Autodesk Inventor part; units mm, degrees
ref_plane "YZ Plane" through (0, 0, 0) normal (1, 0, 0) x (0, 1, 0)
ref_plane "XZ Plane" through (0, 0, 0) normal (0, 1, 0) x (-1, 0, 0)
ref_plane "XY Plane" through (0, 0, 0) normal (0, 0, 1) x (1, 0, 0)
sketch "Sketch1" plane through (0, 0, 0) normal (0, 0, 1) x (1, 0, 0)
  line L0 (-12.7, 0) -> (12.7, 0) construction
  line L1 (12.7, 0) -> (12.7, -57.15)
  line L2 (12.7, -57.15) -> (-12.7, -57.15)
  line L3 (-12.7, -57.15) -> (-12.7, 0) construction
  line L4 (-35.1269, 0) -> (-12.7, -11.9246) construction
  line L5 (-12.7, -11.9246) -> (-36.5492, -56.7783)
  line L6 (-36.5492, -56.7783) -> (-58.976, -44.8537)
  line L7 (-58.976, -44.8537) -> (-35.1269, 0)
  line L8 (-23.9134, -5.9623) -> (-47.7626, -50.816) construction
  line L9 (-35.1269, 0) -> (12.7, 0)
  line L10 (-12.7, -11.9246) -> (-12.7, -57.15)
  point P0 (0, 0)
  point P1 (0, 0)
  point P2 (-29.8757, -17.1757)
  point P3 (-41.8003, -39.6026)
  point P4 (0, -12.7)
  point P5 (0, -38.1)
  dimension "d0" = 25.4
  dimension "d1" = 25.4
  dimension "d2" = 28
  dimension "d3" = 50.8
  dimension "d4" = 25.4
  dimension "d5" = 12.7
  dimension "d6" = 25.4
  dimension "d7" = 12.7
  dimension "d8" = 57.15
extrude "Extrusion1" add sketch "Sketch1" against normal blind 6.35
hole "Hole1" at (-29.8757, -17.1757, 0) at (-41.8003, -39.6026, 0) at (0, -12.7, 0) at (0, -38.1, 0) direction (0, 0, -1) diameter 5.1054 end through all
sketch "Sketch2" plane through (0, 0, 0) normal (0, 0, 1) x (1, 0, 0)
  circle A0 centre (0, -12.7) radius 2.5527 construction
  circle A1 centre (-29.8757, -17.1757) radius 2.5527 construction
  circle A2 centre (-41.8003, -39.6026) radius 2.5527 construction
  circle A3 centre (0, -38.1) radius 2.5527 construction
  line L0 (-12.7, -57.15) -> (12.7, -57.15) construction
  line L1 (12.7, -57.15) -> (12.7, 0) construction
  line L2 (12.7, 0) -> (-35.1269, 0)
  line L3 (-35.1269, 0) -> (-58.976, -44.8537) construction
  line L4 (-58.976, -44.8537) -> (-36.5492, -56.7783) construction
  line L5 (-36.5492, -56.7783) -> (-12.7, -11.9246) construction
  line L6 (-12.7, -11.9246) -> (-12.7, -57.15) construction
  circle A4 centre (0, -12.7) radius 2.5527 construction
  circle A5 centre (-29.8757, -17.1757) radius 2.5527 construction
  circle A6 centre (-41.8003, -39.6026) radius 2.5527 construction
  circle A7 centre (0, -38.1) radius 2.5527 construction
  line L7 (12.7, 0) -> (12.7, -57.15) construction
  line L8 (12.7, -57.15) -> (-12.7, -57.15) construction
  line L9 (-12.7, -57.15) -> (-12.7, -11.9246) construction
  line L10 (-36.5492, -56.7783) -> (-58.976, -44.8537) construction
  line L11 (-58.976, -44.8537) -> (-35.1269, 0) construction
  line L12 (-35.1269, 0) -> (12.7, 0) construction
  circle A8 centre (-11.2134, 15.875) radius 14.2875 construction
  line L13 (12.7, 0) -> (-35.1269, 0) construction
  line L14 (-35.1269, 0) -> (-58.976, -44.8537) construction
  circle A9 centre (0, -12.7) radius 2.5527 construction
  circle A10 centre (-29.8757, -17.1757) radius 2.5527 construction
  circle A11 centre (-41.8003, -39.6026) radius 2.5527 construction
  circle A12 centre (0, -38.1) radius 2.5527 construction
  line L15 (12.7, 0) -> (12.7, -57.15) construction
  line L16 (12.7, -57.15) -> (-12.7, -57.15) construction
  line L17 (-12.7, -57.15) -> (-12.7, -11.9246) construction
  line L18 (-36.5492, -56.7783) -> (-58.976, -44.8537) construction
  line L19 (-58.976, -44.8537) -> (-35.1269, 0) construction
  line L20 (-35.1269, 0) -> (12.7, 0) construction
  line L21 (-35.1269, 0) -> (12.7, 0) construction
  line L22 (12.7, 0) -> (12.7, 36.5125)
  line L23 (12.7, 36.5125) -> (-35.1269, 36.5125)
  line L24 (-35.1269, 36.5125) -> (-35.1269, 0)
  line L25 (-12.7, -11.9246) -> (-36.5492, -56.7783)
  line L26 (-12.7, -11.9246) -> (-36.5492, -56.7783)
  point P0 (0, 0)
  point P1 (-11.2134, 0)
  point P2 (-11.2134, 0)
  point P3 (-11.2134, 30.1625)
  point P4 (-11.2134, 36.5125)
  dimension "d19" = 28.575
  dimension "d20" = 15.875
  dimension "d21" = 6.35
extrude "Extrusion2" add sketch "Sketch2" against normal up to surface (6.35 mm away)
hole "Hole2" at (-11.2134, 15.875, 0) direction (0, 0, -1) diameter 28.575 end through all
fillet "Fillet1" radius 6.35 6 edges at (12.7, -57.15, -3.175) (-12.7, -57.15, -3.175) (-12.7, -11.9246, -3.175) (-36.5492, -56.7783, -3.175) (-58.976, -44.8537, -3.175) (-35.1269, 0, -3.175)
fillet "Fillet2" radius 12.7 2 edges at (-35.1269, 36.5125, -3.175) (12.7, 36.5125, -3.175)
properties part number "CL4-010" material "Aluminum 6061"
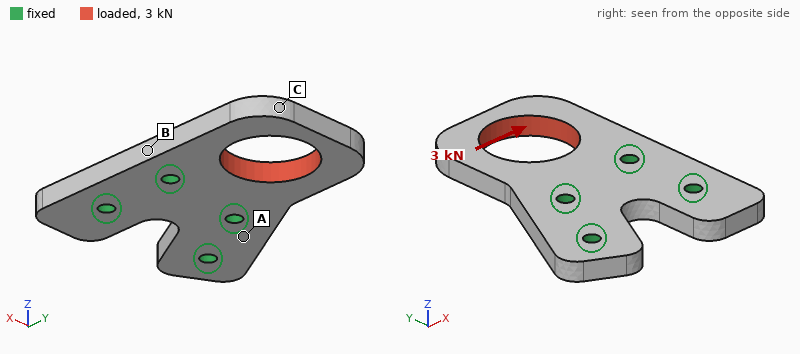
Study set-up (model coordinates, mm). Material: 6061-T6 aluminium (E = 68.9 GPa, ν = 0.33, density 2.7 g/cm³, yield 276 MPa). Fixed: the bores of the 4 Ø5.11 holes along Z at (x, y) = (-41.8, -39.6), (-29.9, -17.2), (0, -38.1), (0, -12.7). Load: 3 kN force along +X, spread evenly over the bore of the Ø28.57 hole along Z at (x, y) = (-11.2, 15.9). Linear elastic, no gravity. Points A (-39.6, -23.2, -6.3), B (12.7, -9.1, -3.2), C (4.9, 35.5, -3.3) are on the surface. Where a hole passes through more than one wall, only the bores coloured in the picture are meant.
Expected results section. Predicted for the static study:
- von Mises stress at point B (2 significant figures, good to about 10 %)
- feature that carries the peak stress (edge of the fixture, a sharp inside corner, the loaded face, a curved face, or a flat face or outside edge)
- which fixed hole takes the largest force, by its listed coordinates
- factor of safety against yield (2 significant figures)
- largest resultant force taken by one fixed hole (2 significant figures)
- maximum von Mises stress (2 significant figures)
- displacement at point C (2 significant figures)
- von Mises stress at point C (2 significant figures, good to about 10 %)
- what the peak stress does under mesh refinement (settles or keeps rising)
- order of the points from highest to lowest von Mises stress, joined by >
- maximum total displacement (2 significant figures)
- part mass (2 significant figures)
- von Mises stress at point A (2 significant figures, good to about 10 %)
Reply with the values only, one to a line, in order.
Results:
42 MPa
the loaded face
(0, -12.7)
3.3
2.7 kN
83 MPa
83 µm
23 MPa
settles
B > C > A
83 µm
67 g
9.7 MPa
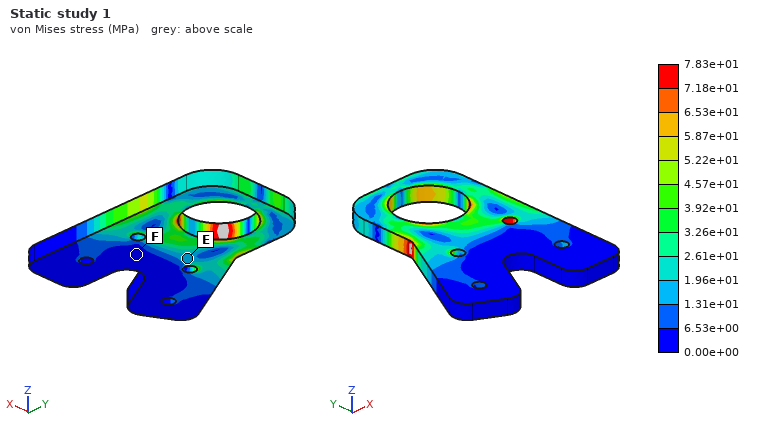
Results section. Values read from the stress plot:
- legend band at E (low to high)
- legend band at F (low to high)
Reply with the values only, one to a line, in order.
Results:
1.31e+01 to 1.96e+01 MPa
0.00e+00 to 6.53e+00 MPa
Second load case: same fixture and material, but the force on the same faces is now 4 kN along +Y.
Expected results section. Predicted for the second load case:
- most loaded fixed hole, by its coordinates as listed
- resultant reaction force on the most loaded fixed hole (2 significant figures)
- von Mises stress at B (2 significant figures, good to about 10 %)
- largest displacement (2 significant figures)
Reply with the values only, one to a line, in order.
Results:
(0, -12.7)
1.9 kN
20 MPa
28 µm
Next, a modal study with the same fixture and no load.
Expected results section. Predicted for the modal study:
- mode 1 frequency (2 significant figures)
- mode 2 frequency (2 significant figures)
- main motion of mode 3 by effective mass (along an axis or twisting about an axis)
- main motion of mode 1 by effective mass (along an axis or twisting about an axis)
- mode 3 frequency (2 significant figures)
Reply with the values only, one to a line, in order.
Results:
2200 Hz
4500 Hz
along X
along Z
7500 Hz
